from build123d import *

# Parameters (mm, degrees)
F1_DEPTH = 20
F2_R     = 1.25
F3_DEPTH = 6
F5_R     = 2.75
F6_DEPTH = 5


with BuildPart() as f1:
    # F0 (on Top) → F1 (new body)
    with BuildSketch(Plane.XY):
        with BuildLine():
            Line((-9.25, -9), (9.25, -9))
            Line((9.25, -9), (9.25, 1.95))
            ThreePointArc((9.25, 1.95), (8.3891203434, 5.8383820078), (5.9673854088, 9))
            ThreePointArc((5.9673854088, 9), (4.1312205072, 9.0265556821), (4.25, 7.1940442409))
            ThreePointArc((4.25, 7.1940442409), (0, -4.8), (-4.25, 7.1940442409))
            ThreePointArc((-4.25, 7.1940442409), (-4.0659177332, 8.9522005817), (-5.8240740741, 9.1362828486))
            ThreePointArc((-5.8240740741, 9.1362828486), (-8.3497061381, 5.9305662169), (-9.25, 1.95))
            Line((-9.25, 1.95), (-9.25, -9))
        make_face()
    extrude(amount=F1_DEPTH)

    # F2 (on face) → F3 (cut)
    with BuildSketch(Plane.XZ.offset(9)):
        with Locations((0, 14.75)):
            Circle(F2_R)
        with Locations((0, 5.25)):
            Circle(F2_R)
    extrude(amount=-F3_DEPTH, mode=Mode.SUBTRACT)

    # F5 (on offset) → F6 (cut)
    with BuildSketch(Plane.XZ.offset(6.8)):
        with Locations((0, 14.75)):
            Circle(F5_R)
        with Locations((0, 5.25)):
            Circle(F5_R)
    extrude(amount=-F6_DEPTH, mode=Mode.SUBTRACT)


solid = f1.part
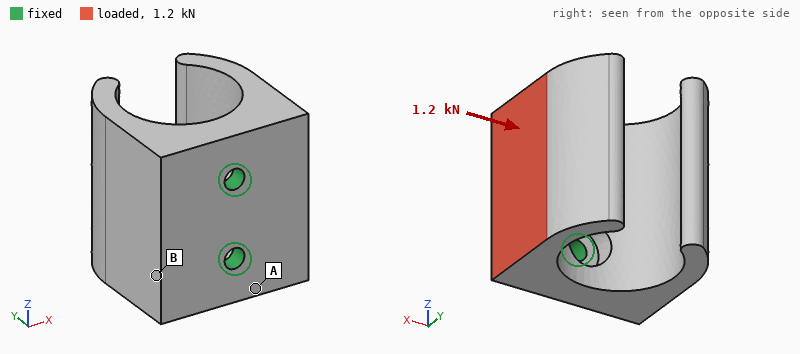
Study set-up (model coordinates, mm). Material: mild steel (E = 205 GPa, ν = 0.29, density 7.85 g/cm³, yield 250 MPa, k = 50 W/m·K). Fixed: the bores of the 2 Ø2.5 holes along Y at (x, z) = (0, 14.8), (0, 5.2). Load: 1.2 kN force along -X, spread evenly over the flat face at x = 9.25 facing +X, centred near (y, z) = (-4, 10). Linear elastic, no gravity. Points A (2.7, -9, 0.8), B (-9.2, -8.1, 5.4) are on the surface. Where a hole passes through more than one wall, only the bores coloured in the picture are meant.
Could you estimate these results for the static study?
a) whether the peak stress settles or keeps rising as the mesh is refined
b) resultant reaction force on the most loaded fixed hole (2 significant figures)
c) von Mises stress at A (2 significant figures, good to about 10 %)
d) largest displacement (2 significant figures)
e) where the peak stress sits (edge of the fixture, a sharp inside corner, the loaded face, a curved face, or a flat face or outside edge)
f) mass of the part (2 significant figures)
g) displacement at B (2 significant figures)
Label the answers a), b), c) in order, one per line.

a) keeps rising
b) 600 N
c) 60 MPa
d) 39 µm
e) edge of the fixture
f) 26 g
g) 9.7 µm
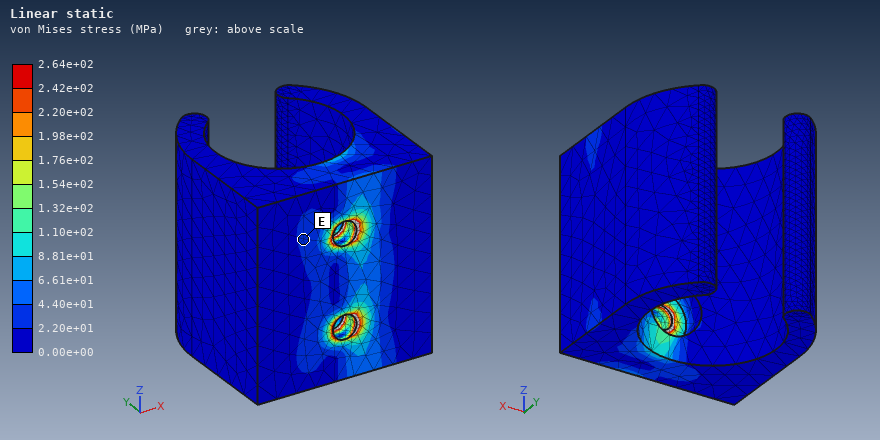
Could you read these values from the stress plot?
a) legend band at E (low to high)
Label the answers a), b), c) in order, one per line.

a) 2.20e+01 to 4.40e+01 MPa
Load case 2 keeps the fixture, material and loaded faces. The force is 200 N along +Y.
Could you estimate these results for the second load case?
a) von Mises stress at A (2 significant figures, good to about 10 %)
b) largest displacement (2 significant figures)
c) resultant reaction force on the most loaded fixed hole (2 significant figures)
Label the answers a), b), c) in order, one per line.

a) 20 MPa
b) 12 µm
c) 100 N
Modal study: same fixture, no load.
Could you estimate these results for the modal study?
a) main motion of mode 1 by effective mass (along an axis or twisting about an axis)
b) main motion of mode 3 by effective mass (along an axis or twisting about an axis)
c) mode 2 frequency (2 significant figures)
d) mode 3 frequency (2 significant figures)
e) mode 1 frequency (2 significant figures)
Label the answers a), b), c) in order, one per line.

a) along X
b) along Z
c) 9600 Hz
d) 13 kHz
e) 5800 Hz
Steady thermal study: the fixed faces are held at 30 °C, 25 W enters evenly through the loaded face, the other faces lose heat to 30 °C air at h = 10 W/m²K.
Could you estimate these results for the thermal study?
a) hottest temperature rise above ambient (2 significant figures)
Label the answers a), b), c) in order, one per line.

a) 65 K
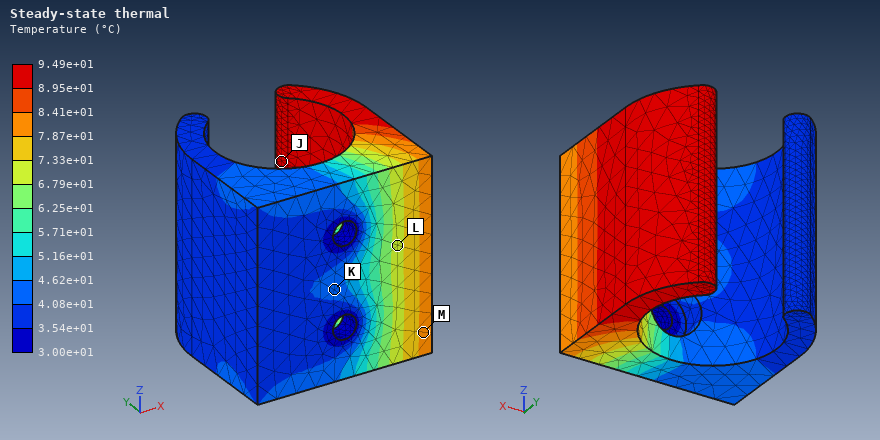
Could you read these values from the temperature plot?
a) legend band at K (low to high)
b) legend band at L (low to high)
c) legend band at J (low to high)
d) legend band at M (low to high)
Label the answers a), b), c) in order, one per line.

a) 4.08e+01 to 4.62e+01 °C
b) 6.79e+01 to 7.33e+01 °C
c) 8.95e+01 to 9.49e+01 °C
d) 7.87e+01 to 8.41e+01 °C
